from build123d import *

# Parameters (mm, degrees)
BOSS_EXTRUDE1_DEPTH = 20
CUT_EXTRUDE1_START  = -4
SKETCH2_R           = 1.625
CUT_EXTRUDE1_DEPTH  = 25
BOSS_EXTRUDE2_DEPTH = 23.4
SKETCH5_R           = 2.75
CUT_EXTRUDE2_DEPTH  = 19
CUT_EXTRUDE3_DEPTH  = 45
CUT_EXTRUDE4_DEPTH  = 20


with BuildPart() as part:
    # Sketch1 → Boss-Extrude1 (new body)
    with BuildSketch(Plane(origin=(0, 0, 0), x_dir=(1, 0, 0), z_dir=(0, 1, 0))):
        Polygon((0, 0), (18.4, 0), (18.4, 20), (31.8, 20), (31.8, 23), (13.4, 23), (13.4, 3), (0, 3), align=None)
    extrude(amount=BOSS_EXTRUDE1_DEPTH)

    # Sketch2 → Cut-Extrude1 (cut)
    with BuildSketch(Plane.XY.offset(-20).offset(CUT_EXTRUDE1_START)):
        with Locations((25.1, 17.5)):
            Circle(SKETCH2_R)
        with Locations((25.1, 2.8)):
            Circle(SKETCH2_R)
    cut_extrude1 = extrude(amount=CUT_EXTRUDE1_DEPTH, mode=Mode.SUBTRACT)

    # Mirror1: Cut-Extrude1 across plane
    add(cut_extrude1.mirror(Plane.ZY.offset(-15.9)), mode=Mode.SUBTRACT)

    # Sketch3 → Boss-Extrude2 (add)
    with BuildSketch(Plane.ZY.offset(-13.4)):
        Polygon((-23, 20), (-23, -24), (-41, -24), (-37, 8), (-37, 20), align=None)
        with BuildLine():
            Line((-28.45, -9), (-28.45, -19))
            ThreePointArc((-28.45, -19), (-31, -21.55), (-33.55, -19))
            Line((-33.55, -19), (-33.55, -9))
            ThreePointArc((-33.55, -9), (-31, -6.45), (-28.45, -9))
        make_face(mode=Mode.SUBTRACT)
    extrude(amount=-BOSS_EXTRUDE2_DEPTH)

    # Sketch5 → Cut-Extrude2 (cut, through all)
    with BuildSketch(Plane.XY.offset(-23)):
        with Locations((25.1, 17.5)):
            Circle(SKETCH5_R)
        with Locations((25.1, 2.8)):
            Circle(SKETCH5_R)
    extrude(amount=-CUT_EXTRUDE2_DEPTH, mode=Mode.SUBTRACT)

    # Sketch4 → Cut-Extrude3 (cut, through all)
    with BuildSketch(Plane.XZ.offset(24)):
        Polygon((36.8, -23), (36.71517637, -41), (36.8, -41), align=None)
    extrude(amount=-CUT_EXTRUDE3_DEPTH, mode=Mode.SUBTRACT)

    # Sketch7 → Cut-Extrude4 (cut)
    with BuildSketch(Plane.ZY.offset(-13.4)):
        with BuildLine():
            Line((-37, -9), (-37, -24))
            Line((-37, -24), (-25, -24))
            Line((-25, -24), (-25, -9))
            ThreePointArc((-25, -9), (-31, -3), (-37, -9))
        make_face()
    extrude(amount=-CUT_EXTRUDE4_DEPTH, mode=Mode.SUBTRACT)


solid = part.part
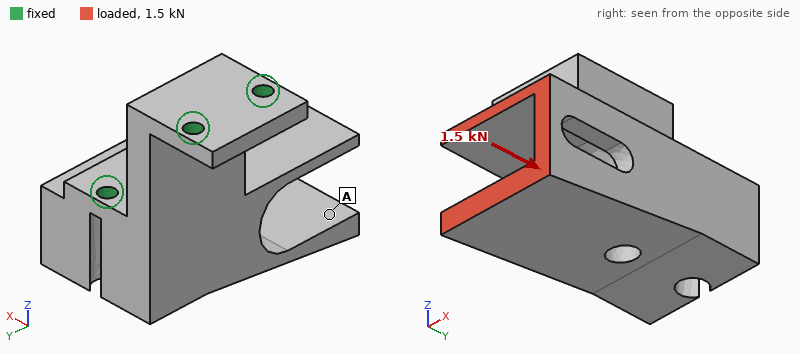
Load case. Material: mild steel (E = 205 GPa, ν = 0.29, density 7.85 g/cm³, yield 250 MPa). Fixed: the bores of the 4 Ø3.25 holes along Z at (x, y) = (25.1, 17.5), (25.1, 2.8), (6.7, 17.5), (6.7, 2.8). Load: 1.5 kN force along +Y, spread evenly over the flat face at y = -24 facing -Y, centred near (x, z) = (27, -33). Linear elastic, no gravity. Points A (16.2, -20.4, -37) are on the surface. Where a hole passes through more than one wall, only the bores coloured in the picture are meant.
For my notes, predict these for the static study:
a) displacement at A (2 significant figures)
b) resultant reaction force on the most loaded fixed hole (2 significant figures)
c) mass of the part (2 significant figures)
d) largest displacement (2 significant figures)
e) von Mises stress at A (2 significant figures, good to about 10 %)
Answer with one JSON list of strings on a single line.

["15 µm", "1.3 kN", "110 g", "20 µm", "10 MPa"]
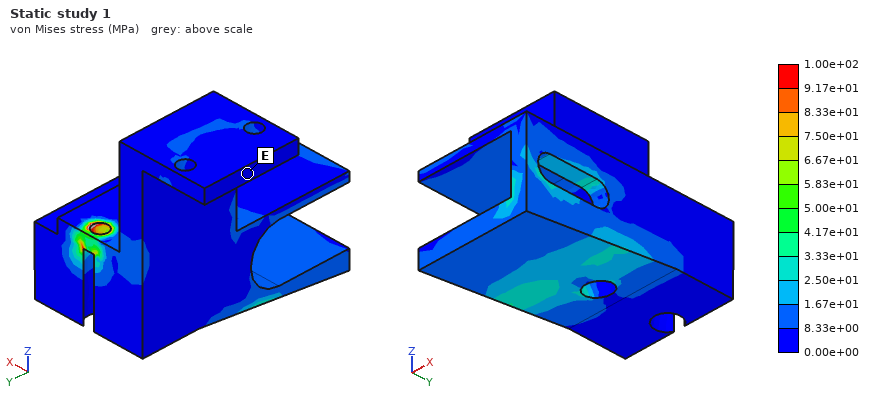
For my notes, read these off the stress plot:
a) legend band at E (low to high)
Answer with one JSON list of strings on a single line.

["0.00e+00 to 8.33e+00 MPa"]
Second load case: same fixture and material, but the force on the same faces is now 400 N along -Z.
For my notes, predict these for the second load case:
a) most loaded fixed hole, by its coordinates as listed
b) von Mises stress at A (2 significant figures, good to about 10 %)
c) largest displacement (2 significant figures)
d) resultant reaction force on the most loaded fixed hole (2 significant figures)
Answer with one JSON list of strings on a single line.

["(25.1, 2.8)", "18 MPa", "46 µm", "930 N"]
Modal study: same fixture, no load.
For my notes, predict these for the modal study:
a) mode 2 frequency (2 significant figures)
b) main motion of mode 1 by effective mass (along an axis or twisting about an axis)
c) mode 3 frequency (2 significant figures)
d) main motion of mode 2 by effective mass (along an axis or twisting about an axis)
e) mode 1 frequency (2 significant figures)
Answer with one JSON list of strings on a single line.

["6000 Hz", "along X", "7900 Hz", "along Z", "5800 Hz"]
